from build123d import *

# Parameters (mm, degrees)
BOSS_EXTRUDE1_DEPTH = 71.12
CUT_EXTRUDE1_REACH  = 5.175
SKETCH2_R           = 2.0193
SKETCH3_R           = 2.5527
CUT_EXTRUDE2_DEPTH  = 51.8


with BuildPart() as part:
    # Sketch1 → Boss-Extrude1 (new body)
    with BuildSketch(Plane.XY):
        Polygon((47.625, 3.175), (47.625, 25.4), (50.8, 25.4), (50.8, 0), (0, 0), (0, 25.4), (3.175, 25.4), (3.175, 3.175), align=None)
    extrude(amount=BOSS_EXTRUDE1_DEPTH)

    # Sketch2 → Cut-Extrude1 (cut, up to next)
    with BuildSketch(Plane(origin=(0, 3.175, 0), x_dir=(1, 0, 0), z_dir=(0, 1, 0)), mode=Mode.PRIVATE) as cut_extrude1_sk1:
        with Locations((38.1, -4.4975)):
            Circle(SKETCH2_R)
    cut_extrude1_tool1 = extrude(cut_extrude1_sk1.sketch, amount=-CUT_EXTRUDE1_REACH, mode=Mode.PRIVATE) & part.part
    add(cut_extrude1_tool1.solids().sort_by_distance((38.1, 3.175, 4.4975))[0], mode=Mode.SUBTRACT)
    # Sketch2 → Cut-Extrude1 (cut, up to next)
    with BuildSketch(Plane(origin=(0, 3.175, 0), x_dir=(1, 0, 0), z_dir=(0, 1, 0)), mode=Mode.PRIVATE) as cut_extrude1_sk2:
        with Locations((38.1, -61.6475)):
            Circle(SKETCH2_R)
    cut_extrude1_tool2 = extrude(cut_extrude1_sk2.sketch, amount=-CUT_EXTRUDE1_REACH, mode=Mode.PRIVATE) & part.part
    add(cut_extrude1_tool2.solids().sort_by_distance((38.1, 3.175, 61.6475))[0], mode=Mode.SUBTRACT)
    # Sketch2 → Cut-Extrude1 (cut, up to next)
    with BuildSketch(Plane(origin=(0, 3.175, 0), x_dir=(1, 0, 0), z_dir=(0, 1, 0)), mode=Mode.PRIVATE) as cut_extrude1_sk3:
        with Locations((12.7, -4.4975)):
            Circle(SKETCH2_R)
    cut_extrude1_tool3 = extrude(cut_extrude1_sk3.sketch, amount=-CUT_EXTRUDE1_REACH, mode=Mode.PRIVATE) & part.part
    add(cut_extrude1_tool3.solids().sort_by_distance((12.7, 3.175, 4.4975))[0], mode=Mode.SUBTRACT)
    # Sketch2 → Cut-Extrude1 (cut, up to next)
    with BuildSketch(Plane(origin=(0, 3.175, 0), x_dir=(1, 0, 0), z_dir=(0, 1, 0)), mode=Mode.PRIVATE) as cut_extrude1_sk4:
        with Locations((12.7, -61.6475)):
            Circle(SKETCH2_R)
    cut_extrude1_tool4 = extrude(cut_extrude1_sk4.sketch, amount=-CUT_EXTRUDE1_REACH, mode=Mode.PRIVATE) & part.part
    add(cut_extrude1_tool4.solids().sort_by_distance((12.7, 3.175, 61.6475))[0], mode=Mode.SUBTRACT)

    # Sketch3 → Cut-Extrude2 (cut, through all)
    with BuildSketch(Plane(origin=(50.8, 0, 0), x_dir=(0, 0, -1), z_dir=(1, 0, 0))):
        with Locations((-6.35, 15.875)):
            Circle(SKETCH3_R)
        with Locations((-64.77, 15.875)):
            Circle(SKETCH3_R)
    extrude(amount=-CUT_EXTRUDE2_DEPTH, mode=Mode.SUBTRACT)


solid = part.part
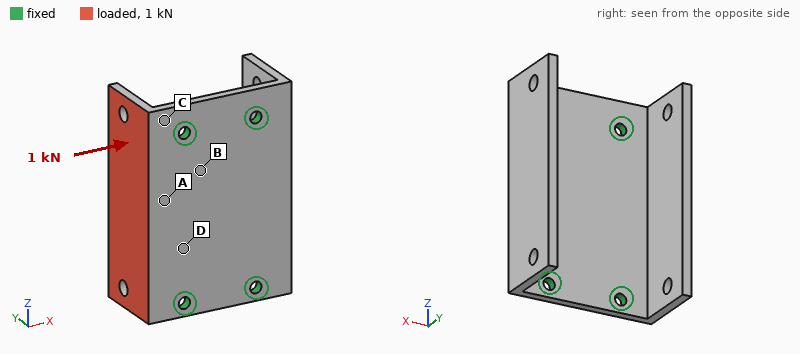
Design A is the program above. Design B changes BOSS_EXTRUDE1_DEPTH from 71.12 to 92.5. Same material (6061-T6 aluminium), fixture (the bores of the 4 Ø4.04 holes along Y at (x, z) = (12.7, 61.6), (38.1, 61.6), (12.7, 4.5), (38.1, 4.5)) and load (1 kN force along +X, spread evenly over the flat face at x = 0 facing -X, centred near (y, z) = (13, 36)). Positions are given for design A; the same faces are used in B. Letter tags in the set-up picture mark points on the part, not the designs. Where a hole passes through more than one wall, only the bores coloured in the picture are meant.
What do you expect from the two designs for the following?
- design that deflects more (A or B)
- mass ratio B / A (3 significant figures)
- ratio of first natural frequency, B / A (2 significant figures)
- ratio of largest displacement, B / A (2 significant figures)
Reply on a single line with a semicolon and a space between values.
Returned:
A; 1.31; 0.96; 0.85
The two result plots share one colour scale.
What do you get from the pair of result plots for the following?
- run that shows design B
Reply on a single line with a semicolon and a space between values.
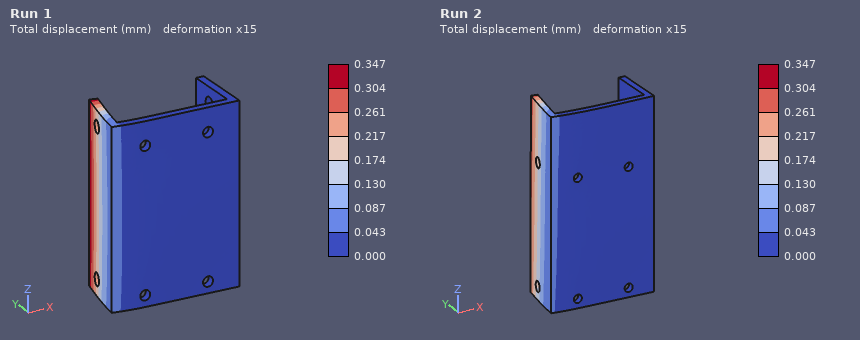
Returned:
Run 2
